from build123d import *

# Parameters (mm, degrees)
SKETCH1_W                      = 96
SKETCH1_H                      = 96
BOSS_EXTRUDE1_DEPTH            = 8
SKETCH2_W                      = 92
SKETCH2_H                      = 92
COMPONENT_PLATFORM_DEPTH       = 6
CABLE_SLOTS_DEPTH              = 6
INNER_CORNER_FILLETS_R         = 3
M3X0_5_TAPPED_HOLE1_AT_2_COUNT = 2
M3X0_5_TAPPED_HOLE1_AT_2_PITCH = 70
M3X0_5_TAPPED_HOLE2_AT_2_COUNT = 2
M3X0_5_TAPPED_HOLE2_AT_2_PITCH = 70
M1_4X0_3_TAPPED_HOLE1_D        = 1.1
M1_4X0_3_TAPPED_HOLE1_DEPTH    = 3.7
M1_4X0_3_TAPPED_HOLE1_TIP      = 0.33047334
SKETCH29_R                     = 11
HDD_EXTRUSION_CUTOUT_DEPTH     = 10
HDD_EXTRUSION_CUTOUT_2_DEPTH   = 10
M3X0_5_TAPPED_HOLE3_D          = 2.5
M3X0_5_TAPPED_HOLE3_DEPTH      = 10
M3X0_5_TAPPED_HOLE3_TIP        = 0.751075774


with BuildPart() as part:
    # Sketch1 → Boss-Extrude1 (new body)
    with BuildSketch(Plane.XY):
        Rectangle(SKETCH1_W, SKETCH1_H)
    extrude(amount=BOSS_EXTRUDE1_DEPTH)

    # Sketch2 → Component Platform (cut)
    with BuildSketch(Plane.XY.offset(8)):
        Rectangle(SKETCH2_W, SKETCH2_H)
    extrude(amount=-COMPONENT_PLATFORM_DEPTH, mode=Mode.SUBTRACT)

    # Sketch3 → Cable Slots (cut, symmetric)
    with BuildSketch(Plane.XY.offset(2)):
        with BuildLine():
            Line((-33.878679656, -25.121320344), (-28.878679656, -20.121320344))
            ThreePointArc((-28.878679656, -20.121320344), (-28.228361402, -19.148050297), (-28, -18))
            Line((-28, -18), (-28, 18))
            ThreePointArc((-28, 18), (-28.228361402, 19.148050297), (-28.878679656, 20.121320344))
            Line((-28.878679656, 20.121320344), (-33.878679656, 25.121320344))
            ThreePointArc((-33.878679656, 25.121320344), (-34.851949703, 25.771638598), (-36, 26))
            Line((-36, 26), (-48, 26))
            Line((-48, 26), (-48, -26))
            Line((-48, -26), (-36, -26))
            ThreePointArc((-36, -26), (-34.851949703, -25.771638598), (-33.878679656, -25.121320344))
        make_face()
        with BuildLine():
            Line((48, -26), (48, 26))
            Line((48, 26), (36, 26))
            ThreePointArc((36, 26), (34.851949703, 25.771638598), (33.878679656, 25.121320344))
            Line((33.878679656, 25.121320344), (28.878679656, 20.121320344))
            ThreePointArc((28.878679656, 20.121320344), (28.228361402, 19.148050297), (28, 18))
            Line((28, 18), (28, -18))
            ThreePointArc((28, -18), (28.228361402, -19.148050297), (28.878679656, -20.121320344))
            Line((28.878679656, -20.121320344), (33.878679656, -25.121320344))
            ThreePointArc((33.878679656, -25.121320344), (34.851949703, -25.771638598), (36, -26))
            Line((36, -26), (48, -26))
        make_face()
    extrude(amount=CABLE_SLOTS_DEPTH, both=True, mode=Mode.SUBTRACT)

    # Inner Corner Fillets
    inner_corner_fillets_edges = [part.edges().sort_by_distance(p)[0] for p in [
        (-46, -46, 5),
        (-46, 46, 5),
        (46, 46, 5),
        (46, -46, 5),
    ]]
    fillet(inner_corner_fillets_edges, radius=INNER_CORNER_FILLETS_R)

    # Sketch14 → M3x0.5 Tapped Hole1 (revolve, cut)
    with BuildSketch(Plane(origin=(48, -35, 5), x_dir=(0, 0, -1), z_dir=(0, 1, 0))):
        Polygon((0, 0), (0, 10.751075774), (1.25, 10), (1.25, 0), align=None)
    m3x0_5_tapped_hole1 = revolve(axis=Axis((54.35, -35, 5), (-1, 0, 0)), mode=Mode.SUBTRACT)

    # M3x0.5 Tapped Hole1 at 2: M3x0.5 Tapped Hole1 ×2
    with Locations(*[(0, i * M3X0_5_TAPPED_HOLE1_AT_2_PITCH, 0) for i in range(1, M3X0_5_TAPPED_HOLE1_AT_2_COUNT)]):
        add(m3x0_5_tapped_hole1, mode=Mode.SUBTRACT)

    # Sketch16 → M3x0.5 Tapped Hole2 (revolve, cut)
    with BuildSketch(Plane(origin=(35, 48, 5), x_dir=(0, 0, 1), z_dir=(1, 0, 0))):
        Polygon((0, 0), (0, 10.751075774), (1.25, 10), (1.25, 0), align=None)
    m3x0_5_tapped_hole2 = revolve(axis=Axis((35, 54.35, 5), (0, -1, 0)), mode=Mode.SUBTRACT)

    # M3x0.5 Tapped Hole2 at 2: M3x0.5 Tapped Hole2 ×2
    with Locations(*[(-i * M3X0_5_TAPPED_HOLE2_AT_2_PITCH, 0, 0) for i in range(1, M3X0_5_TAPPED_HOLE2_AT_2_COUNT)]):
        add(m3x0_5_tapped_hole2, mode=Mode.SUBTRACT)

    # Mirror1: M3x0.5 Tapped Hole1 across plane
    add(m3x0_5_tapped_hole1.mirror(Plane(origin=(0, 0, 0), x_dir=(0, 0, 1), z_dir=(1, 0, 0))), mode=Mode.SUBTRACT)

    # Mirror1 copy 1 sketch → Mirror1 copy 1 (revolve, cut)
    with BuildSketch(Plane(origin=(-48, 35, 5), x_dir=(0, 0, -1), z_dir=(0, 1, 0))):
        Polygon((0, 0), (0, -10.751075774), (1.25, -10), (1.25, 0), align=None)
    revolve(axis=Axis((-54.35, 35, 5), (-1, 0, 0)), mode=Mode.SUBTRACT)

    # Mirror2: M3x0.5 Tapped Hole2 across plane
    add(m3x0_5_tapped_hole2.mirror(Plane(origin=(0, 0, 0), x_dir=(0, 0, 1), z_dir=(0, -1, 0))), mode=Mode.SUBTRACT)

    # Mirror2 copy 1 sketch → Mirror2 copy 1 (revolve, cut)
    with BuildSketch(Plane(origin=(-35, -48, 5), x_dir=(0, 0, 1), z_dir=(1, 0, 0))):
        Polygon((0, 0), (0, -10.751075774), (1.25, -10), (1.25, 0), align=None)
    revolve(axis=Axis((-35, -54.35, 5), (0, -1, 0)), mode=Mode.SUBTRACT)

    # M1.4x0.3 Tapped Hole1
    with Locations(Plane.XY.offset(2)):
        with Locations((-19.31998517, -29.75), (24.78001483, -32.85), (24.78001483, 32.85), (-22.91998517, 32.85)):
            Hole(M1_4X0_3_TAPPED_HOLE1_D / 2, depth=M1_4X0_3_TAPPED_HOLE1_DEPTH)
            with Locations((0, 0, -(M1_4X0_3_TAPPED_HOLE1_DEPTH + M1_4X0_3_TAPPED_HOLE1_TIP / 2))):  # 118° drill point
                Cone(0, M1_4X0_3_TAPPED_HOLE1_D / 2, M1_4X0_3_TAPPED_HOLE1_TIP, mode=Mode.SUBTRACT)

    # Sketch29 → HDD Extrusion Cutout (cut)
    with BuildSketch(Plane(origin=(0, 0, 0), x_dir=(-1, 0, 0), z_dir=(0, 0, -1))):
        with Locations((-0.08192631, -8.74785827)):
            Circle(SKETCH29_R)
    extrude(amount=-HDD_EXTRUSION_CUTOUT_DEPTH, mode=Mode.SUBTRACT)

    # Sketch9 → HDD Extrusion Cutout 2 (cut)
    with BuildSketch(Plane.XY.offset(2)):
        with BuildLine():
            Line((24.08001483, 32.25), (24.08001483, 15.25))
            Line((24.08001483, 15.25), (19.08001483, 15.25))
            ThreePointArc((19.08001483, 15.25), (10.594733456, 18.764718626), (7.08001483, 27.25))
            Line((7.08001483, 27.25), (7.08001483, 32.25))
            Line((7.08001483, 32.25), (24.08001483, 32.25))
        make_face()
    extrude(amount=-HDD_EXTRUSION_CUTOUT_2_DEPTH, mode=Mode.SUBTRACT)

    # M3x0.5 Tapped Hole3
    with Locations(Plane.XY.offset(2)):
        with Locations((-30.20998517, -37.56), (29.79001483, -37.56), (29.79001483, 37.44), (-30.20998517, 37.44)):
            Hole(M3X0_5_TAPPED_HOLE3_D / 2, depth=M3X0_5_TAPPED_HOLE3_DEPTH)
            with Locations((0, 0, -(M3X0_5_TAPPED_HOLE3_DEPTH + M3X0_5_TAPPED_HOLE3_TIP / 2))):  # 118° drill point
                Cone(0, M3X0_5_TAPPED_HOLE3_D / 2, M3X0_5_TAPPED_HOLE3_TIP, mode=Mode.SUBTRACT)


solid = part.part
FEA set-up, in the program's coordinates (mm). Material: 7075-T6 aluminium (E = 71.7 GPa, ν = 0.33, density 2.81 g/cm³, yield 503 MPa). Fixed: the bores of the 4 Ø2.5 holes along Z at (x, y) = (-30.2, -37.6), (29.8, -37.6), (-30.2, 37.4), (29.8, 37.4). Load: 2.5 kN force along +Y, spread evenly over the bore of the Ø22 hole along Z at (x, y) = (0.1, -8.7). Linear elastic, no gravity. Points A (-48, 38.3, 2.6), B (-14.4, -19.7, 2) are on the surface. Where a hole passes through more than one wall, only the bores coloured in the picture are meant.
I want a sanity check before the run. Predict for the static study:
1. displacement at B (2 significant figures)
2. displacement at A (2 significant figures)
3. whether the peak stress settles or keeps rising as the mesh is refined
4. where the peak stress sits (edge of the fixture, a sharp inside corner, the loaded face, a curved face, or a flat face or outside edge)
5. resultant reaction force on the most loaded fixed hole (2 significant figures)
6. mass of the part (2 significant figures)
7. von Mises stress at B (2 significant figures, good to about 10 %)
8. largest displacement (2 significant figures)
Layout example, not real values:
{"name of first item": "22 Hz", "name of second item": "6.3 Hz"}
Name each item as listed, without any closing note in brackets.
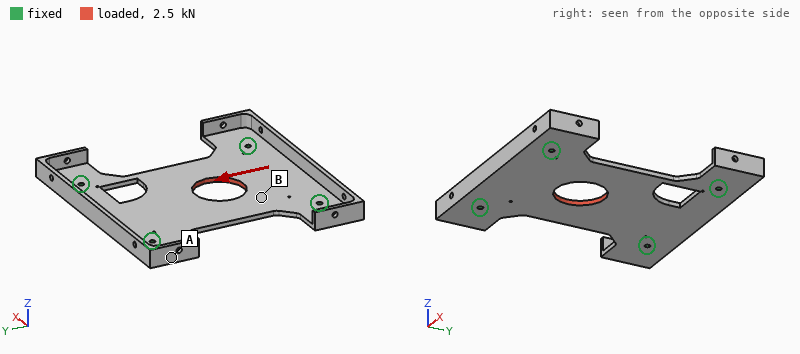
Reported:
{"displacement at B": "12 µm", "displacement at A": "4.8 µm", "whether the peak stress settles or keeps rising as the mesh is refined": "keeps rising", "where the peak stress sits": "edge of the fixture", "resultant reaction force on the most loaded fixed hole": "840 N", "mass of the part": "46 g", "von Mises stress at B": "16 MPa", "largest displacement": "23 µm"}
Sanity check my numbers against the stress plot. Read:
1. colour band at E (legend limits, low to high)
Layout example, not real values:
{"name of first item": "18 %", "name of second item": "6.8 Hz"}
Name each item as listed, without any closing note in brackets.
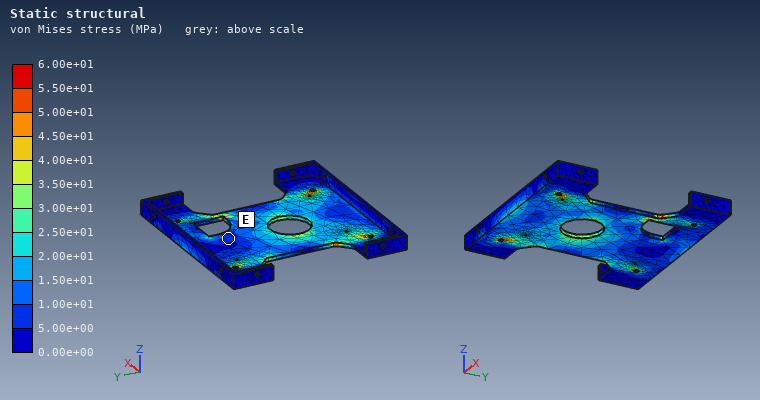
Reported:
{"colour band at E": "5.00e+00 to 1.00e+01 MPa"}
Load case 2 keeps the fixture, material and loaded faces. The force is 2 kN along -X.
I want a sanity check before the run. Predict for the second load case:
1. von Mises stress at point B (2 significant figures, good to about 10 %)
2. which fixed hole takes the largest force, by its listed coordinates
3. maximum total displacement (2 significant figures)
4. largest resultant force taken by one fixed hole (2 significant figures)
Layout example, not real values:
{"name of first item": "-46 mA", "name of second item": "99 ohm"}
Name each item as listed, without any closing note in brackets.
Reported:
{"von Mises stress at point B": "19 MPa", "which fixed hole takes the largest force, by its listed coordinates": "(-30.2, -37.6)", "maximum total displacement": "19 µm", "largest resultant force taken by one fixed hole": "810 N"}
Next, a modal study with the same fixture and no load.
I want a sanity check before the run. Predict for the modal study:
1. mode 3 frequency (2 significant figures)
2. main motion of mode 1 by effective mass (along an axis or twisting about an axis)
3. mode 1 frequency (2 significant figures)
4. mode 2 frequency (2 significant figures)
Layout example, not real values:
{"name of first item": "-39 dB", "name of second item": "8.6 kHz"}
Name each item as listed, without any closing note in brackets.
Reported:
{"mode 3 frequency": "3300 Hz", "main motion of mode 1 by effective mass": "along Z", "mode 1 frequency": "1500 Hz", "mode 2 frequency": "2500 Hz"}
